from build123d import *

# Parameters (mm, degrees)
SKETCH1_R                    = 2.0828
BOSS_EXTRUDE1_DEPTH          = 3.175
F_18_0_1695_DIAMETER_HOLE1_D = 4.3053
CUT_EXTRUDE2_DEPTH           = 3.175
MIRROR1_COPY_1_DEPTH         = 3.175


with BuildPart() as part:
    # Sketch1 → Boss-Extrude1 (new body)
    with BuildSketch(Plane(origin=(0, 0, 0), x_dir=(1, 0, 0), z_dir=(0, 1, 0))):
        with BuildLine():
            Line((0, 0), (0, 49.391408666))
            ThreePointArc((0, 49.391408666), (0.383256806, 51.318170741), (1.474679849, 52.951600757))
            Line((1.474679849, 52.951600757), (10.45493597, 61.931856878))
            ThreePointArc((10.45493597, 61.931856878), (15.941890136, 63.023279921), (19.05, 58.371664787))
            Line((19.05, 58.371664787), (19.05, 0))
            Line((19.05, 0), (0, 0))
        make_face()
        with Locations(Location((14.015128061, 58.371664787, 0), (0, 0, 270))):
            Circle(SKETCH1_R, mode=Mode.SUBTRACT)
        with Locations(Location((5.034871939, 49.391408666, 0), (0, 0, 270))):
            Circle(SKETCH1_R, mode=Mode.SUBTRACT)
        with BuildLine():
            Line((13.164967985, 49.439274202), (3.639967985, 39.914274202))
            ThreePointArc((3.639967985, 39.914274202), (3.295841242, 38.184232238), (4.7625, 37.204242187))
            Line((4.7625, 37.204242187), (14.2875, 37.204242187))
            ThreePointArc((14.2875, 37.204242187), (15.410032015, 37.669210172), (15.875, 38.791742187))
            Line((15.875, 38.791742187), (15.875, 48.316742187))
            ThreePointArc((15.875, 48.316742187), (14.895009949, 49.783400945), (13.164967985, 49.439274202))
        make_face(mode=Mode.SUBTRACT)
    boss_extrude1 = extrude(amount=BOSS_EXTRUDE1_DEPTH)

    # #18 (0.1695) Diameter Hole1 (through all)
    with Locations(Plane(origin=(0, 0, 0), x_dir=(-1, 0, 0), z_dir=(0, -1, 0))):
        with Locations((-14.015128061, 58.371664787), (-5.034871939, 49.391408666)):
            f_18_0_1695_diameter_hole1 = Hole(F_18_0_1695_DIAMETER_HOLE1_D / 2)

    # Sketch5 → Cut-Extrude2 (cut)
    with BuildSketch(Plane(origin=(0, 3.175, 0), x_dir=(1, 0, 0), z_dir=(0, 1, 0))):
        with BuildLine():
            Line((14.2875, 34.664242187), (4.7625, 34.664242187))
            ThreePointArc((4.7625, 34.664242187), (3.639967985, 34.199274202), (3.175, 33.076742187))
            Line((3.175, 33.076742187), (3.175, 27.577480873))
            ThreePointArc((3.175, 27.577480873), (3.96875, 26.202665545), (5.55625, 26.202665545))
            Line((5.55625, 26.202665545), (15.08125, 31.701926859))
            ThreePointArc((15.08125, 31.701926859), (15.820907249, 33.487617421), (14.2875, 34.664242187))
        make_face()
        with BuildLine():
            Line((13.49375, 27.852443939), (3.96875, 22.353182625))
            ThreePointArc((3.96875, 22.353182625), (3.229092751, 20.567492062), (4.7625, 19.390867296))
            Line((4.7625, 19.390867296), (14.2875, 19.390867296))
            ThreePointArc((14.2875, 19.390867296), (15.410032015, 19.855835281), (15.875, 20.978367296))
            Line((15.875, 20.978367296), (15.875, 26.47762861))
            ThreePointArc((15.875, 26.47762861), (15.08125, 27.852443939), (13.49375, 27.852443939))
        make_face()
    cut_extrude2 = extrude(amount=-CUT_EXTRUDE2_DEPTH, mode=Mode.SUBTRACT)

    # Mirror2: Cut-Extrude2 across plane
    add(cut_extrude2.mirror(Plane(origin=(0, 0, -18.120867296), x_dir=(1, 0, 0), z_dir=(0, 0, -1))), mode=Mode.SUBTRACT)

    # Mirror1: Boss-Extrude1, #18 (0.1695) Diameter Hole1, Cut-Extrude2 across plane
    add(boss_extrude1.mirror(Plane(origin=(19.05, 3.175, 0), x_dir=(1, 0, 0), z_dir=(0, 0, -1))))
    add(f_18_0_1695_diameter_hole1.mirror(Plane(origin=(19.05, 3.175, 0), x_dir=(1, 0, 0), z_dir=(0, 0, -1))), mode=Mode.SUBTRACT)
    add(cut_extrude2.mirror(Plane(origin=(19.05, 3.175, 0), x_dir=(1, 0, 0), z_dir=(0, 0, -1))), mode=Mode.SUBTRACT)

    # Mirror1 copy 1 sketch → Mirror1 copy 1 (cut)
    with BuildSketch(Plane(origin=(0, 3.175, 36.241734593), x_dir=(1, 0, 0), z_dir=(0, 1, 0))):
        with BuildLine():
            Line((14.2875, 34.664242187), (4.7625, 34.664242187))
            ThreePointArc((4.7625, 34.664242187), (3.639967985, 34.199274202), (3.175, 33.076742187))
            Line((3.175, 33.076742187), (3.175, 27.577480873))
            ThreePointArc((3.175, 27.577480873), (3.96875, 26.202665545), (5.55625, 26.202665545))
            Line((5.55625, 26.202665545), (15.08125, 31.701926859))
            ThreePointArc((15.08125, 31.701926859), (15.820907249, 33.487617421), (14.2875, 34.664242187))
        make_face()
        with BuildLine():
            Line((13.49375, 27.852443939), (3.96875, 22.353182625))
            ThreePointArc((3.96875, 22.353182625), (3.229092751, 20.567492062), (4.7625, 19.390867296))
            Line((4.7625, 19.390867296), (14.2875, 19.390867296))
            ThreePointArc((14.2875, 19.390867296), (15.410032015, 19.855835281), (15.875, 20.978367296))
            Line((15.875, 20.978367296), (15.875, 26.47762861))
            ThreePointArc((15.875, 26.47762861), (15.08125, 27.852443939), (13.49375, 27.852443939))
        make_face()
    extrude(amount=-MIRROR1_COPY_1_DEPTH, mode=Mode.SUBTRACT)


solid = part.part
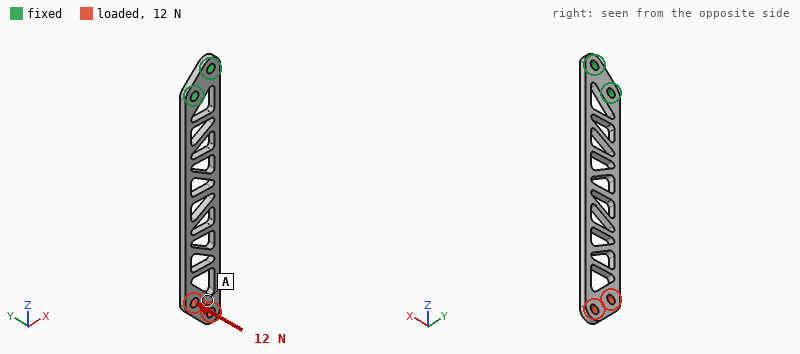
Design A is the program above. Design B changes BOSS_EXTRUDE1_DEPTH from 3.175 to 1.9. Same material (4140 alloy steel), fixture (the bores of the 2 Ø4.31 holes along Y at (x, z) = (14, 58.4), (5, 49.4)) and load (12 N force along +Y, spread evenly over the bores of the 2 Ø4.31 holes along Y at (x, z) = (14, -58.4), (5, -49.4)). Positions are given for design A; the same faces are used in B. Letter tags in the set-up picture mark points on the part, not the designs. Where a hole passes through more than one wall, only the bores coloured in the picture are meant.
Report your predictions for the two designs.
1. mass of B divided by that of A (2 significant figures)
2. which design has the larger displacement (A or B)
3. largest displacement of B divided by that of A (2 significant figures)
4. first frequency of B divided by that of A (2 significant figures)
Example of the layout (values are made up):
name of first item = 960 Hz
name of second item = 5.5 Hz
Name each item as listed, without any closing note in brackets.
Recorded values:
mass of B divided by that of A = 0.60
which design has the larger displacement = B
largest displacement of B divided by that of A = 4.5
first frequency of B divided by that of A = 0.61
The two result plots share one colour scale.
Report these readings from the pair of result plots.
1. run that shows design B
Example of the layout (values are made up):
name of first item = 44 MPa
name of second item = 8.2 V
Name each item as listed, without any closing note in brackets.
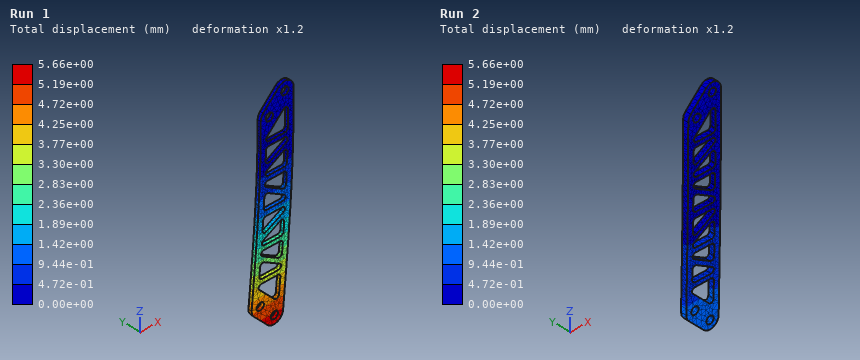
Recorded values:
run that shows design B = Run 1
